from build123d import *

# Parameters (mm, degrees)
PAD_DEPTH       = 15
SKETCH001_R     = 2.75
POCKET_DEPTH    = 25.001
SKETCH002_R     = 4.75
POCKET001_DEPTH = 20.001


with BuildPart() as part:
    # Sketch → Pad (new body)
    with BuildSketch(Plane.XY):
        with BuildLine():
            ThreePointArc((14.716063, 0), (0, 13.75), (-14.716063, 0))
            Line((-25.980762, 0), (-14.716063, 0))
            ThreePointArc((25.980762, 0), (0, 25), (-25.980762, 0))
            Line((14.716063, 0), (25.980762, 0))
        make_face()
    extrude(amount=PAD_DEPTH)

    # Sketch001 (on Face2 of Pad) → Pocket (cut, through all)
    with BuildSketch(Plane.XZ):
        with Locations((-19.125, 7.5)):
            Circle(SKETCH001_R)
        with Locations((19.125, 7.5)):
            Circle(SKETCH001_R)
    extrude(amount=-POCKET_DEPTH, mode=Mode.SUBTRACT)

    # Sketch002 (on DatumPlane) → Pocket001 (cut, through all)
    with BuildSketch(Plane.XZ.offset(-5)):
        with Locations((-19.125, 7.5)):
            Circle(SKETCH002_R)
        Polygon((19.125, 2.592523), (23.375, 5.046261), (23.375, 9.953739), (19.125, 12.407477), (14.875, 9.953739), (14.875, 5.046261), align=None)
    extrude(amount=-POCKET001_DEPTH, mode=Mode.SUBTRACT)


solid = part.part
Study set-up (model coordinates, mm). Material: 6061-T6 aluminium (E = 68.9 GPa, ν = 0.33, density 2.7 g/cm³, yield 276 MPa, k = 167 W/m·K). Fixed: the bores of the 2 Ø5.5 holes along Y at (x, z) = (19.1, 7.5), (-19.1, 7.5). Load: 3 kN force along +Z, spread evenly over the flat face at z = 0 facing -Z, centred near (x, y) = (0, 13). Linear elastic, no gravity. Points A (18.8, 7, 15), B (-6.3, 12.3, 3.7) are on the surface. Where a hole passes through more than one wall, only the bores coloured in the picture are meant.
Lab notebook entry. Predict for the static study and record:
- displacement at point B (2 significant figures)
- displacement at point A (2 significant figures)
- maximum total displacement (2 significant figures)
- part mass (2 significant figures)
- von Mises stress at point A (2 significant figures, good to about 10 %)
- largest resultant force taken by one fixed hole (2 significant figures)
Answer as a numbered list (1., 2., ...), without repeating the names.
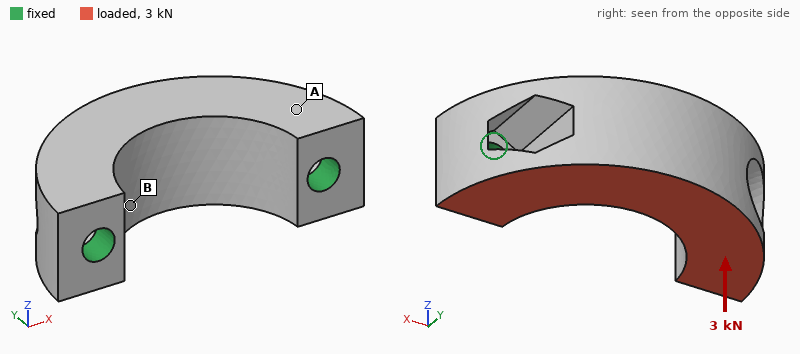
1. 33 µm
2. 17 µm
3. 66 µm
4. 24 g
5. 39 MPa
6. 1.5 kN
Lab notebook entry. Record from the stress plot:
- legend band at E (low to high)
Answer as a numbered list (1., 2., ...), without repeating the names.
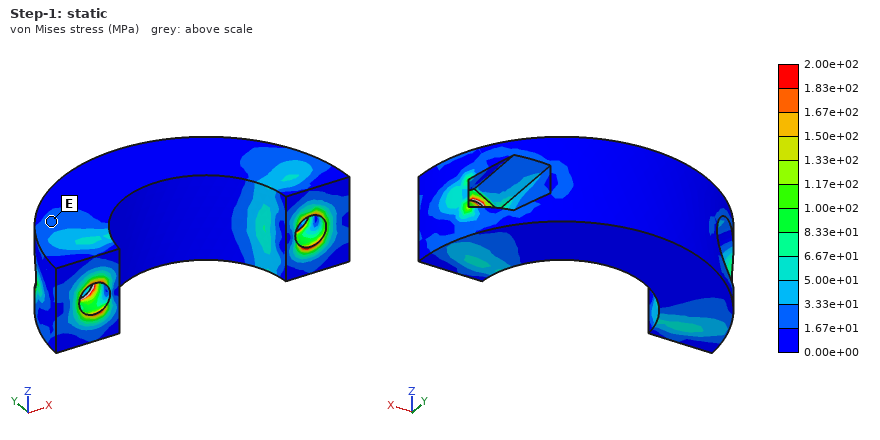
1. 1.67e+01 to 3.33e+01 MPa
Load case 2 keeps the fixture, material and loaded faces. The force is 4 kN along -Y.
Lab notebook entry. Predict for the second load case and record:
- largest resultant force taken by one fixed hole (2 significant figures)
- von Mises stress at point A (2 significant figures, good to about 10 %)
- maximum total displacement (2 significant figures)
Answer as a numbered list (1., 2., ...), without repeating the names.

1. 2.1 kN
2. 28 MPa
3. 59 µm
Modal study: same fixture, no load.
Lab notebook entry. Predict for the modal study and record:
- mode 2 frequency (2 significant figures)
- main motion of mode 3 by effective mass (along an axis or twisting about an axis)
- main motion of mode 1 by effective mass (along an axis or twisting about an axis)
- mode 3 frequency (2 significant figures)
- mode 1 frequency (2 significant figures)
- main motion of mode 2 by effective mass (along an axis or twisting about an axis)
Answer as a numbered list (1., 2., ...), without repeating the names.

1. 17 kHz
2. twisting about Y
3. along Z
4. 20 kHz
5. 8100 Hz
6. along X
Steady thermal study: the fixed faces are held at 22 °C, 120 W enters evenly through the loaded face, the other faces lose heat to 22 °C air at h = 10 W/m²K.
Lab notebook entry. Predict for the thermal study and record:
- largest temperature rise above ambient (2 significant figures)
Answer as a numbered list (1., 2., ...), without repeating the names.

1. 49 K
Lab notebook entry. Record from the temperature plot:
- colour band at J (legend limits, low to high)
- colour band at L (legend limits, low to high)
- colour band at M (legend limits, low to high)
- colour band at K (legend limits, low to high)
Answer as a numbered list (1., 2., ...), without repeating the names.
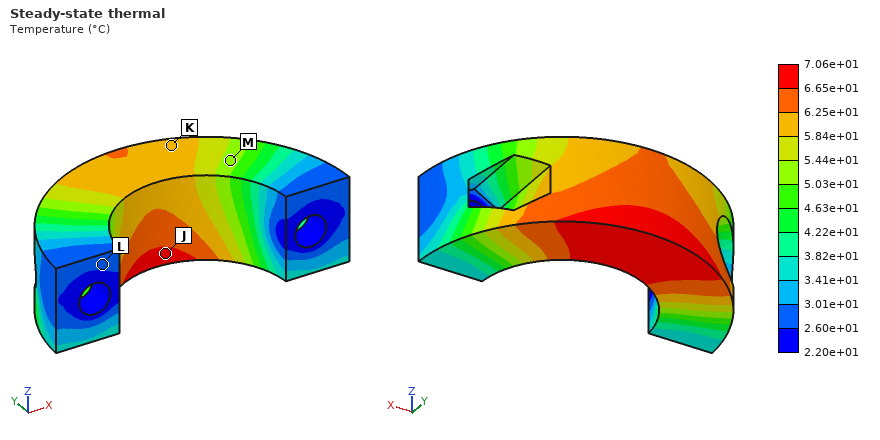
1. 6.65e+01 to 7.06e+01 °C
2. 2.60e+01 to 3.01e+01 °C
3. 5.03e+01 to 5.44e+01 °C
4. 5.84e+01 to 6.25e+01 °C
